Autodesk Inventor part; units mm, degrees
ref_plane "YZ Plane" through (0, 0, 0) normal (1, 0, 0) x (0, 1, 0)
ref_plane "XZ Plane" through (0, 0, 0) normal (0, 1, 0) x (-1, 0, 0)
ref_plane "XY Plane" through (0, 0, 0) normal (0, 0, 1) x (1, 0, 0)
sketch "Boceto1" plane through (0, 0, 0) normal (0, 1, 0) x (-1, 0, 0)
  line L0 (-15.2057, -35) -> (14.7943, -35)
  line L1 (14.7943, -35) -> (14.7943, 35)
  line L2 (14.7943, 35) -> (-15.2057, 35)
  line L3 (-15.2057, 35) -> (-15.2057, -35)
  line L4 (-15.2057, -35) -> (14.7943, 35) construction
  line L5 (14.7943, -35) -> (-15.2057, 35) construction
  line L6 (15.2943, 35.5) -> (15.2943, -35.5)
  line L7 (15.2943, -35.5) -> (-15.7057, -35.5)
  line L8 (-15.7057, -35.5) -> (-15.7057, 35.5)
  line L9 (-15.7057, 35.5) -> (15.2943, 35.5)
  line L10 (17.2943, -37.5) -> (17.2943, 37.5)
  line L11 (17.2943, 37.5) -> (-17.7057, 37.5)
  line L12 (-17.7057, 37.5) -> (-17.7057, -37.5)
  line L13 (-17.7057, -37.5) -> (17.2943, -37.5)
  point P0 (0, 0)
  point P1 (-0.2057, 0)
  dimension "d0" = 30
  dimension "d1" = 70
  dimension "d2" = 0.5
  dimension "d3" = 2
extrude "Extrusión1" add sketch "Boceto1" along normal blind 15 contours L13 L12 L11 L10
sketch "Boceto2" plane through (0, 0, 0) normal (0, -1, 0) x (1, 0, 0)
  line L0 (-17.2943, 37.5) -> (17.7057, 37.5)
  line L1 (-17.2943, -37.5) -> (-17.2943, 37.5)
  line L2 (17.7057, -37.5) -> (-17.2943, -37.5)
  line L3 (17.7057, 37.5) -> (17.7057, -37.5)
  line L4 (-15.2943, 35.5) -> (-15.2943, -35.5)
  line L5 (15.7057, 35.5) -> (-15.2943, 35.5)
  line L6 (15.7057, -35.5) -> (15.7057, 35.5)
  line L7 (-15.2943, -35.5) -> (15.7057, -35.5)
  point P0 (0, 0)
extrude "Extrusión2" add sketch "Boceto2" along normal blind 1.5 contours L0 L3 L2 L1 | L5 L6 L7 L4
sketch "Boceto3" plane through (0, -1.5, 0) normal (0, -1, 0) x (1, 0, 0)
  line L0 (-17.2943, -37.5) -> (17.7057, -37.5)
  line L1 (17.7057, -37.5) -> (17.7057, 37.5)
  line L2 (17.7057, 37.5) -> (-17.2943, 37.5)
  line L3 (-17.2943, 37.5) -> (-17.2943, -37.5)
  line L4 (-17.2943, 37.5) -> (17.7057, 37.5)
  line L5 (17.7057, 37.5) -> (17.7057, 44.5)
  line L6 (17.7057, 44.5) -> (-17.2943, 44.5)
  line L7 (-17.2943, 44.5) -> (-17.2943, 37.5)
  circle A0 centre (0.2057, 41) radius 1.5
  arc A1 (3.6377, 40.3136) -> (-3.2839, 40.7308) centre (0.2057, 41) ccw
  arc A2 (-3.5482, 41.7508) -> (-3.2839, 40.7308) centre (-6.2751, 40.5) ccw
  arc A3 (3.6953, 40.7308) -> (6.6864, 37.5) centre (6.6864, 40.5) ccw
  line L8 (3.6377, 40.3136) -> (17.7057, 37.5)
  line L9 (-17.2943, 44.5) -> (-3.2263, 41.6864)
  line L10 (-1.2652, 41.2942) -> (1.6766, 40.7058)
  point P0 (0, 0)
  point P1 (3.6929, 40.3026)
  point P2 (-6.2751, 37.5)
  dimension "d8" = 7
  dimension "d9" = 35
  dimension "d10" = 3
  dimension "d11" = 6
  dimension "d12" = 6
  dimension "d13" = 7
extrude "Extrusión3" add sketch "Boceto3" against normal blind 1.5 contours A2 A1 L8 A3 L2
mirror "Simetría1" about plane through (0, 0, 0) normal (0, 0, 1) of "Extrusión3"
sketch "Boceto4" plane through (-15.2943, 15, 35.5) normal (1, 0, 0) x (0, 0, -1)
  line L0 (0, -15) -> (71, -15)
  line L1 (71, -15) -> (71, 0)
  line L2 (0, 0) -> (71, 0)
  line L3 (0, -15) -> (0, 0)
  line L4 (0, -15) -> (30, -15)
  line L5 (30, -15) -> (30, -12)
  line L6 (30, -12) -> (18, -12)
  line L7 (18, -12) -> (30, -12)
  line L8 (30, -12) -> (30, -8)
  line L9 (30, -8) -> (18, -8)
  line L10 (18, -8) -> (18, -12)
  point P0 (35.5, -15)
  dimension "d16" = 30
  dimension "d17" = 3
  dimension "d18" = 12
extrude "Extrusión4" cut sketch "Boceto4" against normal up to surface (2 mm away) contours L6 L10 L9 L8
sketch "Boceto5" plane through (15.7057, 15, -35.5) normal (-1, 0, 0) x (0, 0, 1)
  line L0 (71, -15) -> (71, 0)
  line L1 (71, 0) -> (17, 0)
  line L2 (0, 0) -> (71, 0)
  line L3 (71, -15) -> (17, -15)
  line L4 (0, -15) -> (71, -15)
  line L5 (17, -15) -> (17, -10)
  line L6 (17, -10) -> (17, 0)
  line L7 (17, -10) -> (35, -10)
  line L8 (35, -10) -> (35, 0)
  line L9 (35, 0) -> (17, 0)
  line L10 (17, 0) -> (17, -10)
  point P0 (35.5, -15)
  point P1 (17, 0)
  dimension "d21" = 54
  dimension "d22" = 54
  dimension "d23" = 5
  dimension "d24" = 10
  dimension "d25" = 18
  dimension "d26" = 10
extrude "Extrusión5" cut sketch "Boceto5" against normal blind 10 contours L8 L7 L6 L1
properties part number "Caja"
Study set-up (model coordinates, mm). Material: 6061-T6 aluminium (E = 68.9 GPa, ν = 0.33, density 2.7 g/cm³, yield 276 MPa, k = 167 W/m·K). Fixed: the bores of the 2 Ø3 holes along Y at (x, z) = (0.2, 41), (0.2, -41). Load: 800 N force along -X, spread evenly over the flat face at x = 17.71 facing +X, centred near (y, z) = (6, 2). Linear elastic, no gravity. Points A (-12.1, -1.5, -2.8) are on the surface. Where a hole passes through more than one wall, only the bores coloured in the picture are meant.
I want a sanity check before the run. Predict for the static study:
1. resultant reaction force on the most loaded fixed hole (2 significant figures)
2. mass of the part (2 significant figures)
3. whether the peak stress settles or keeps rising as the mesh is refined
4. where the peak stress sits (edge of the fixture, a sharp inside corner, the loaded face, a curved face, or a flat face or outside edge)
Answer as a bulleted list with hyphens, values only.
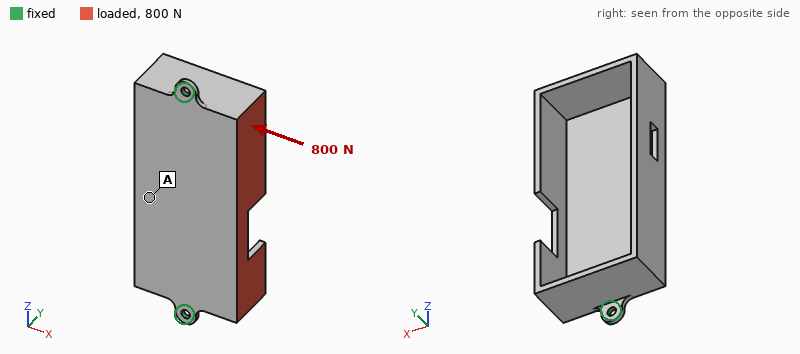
- 420 N
- 27 g
- keeps rising
- edge of the fixture
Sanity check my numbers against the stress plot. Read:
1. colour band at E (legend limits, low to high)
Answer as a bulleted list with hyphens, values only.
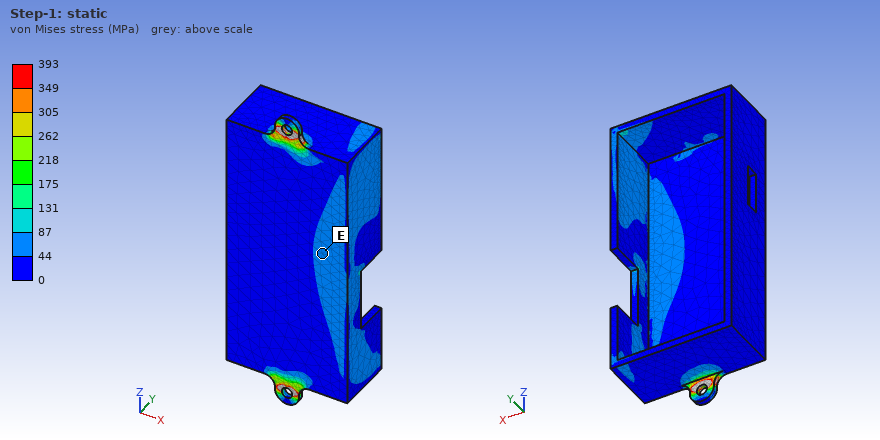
- 44 to 87 MPa
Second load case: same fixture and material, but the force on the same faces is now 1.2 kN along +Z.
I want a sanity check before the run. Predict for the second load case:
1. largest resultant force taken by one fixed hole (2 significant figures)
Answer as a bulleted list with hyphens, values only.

- 670 N
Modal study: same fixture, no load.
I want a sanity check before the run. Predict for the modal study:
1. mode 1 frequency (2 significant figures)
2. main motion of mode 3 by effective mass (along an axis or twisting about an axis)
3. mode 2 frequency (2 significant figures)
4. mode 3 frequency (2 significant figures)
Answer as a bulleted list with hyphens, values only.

- 1000 Hz
- along Y
- 2100 Hz
- 2800 Hz
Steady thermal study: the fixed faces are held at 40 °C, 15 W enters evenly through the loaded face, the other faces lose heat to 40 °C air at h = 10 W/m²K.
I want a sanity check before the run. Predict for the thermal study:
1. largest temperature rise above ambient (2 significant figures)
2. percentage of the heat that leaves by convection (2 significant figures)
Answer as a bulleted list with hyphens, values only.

- 32 K
- 14 %
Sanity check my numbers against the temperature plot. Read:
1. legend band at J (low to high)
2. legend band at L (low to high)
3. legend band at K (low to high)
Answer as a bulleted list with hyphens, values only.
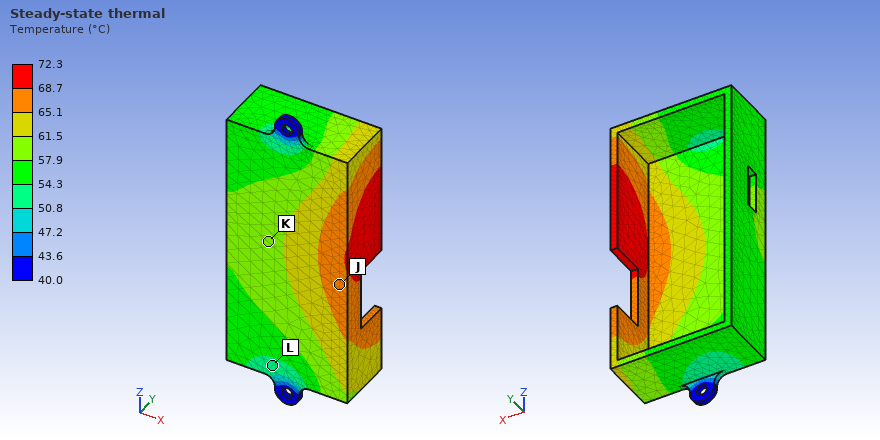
- 65.1 to 68.7 °C
- 50.8 to 54.3 °C
- 57.9 to 61.5 °C
